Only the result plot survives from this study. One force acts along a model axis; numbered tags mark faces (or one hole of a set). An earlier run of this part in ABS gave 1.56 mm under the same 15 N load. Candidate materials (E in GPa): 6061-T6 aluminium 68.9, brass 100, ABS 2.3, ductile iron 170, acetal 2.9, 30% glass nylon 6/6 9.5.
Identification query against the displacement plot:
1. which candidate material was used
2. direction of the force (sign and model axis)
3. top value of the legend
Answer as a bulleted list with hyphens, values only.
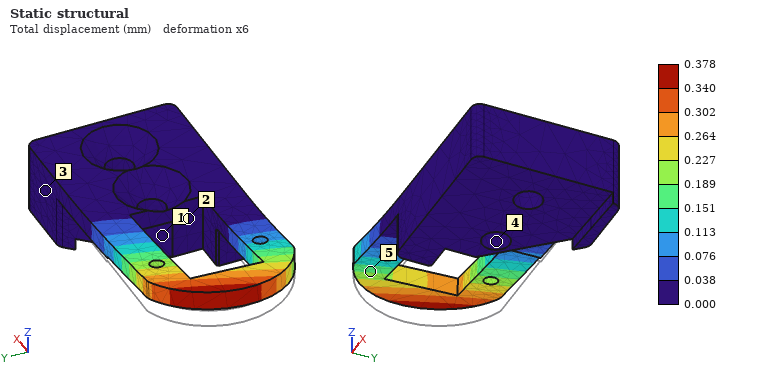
- 30% glass nylon 6/6
- +Z
- 0.378 mm
